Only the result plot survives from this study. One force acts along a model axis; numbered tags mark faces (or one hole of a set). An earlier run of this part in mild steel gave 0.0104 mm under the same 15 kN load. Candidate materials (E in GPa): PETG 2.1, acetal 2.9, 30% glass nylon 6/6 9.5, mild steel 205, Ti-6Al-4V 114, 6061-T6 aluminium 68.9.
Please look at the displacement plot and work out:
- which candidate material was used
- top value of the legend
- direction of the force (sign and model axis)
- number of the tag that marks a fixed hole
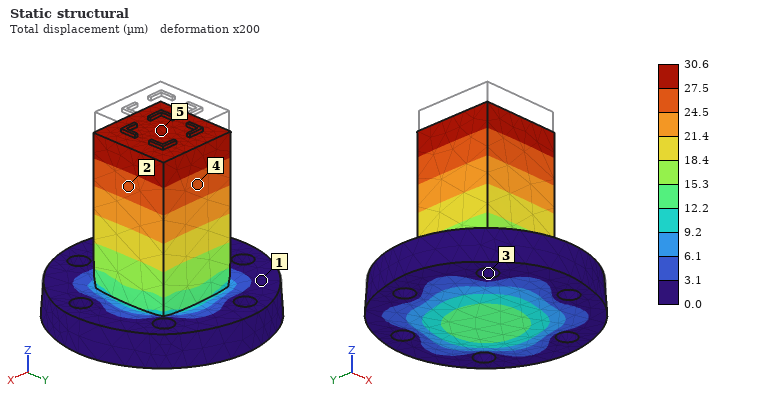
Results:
6061-T6 aluminium
30.6 µm
-Z
3
